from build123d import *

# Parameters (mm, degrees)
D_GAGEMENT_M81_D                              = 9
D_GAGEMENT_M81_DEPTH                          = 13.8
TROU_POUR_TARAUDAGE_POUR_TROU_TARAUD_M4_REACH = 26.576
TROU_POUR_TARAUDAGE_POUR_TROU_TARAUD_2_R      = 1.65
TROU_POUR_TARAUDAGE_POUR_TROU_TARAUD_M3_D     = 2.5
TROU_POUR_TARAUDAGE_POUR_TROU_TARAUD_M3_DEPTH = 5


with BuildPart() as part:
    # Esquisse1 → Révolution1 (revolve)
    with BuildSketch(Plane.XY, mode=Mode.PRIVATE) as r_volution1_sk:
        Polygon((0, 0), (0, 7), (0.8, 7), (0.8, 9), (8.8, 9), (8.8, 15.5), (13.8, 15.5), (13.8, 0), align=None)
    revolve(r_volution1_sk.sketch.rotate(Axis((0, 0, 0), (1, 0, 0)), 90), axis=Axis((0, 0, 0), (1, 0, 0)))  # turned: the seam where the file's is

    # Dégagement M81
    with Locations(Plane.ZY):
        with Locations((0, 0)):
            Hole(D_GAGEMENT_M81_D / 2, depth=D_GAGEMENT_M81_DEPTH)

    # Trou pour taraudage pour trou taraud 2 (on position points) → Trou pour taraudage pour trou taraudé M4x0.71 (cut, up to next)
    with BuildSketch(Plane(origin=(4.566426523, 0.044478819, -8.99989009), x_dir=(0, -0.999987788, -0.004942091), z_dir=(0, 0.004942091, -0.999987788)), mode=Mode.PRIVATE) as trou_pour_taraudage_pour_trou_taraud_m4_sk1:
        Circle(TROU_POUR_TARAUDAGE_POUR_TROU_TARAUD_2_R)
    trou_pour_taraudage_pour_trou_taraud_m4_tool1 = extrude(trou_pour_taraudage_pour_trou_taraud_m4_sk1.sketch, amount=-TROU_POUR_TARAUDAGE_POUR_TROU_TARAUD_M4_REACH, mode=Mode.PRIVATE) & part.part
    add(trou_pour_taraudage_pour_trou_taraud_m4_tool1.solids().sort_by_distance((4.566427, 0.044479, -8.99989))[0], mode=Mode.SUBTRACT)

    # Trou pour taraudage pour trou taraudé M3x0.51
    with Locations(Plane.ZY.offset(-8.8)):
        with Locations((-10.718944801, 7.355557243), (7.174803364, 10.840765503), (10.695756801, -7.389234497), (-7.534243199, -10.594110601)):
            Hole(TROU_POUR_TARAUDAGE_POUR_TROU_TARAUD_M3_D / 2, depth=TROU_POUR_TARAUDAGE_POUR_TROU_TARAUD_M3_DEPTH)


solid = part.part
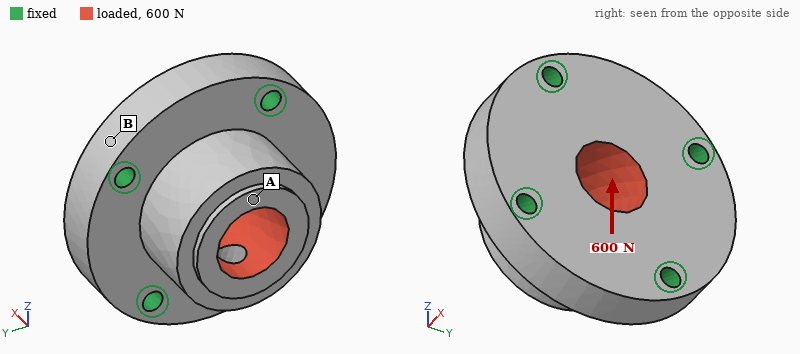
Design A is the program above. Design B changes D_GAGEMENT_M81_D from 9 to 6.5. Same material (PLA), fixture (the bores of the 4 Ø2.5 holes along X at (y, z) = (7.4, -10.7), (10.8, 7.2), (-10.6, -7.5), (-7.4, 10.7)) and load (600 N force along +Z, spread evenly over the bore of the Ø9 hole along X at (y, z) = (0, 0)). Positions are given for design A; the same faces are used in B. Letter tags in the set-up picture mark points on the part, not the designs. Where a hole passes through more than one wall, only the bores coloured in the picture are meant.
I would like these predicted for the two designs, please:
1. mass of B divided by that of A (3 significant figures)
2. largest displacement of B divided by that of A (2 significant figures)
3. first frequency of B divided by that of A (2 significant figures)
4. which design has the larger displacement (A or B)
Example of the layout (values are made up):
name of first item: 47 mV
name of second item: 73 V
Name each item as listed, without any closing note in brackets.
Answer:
mass of B divided by that of A: 1.08
largest displacement of B divided by that of A: 0.91
first frequency of B divided by that of A: 0.97
which design has the larger displacement: A
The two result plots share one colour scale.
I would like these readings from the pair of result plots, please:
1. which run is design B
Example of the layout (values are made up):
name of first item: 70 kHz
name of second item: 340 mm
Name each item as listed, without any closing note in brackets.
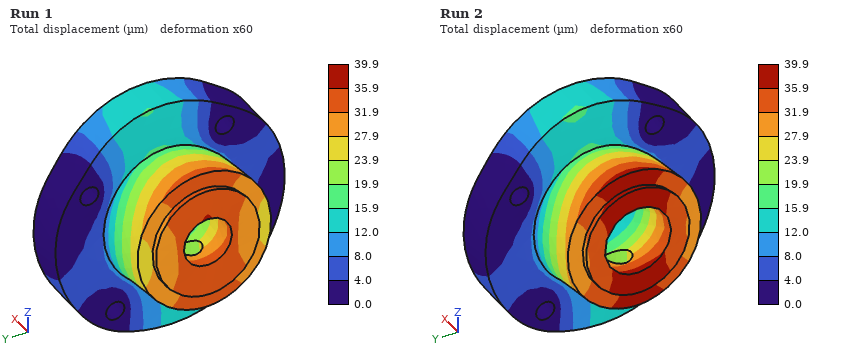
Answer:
which run is design B: Run 1
